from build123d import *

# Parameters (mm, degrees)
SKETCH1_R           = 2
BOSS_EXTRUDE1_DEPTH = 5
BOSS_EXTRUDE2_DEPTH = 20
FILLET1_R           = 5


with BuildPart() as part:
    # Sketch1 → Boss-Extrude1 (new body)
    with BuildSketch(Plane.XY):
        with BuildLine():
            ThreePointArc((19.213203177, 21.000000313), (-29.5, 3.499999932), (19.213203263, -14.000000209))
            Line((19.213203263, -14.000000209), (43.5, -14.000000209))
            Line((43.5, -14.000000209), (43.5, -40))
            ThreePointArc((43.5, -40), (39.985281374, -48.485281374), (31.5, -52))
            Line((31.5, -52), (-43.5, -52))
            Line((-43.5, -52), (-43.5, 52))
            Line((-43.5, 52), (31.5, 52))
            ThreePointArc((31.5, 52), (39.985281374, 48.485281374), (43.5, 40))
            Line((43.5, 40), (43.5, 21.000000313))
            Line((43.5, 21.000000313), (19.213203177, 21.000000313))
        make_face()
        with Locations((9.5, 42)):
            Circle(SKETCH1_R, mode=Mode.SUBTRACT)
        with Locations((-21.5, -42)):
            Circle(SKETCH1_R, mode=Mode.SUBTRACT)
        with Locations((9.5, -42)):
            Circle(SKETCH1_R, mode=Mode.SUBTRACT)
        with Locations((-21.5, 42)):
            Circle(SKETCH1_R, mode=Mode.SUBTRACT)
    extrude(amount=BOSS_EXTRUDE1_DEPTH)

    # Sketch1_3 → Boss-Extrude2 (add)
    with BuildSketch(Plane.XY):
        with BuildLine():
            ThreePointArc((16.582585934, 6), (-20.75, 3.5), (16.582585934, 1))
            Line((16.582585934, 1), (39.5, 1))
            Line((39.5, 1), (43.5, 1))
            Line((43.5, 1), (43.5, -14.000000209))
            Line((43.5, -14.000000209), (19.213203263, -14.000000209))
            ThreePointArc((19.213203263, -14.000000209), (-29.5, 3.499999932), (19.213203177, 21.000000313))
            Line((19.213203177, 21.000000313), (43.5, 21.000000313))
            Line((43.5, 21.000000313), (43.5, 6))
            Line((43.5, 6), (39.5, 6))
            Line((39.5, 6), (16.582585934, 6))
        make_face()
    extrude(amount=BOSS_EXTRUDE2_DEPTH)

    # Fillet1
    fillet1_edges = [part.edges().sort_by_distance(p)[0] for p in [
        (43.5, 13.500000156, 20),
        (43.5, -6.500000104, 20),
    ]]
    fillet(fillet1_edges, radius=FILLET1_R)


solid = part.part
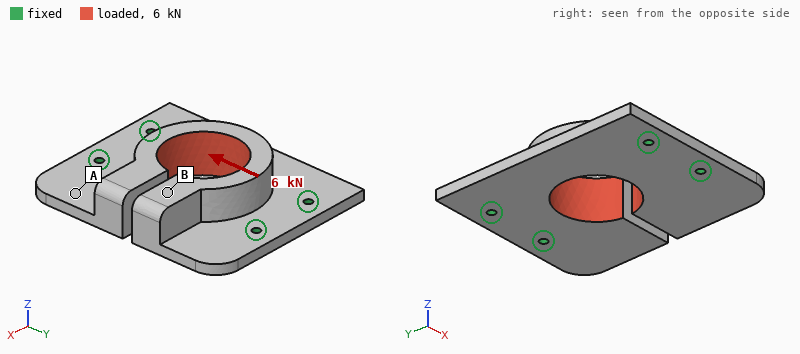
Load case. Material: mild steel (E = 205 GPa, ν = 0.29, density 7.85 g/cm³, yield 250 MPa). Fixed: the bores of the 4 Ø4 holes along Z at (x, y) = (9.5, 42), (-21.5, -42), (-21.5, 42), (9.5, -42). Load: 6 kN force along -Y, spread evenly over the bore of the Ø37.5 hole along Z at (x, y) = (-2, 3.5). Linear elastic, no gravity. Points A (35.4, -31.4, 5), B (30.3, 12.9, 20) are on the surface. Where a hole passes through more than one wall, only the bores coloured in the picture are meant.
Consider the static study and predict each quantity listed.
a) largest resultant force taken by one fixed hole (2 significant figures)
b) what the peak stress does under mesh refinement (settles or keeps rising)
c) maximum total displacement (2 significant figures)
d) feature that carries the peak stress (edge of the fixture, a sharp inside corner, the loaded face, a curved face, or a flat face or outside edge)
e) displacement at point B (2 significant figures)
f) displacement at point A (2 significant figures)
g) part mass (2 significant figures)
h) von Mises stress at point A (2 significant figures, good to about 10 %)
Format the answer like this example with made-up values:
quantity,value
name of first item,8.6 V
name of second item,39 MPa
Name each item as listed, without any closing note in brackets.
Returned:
quantity,value
largest resultant force taken by one fixed hole,1.6 kN
what the peak stress does under mesh refinement,keeps rising
maximum total displacement,43 µm
feature that carries the peak stress,edge of the fixture
displacement at point B,31 µm
displacement at point A,9.8 µm
part mass,520 g
von Mises stress at point A,10 MPa
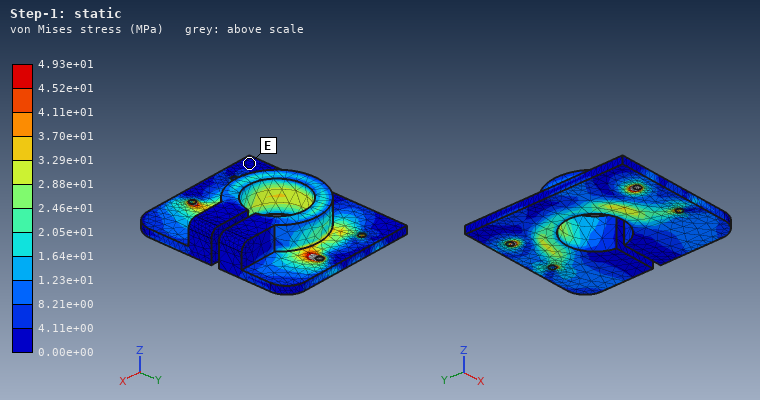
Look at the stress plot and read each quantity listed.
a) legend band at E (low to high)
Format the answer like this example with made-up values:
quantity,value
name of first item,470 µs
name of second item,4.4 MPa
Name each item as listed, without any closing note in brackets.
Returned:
quantity,value
legend band at E,0.00e+00 to 4.11e+00 MPa
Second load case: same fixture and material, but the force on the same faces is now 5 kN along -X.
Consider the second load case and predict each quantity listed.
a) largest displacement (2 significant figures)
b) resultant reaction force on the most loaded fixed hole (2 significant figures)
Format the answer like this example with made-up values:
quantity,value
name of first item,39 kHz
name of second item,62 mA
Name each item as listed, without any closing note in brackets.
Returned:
quantity,value
largest displacement,35 µm
resultant reaction force on the most loaded fixed hole,2.2 kN
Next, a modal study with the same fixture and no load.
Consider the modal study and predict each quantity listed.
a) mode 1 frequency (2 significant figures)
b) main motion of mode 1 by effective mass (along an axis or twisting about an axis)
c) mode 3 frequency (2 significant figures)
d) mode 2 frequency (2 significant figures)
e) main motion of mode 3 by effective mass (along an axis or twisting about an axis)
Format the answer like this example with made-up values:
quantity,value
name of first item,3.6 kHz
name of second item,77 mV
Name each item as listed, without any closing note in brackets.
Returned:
quantity,value
mode 1 frequency,1700 Hz
main motion of mode 1 by effective mass,along Z
mode 3 frequency,3300 Hz
mode 2 frequency,2000 Hz
main motion of mode 3 by effective mass,along Z
